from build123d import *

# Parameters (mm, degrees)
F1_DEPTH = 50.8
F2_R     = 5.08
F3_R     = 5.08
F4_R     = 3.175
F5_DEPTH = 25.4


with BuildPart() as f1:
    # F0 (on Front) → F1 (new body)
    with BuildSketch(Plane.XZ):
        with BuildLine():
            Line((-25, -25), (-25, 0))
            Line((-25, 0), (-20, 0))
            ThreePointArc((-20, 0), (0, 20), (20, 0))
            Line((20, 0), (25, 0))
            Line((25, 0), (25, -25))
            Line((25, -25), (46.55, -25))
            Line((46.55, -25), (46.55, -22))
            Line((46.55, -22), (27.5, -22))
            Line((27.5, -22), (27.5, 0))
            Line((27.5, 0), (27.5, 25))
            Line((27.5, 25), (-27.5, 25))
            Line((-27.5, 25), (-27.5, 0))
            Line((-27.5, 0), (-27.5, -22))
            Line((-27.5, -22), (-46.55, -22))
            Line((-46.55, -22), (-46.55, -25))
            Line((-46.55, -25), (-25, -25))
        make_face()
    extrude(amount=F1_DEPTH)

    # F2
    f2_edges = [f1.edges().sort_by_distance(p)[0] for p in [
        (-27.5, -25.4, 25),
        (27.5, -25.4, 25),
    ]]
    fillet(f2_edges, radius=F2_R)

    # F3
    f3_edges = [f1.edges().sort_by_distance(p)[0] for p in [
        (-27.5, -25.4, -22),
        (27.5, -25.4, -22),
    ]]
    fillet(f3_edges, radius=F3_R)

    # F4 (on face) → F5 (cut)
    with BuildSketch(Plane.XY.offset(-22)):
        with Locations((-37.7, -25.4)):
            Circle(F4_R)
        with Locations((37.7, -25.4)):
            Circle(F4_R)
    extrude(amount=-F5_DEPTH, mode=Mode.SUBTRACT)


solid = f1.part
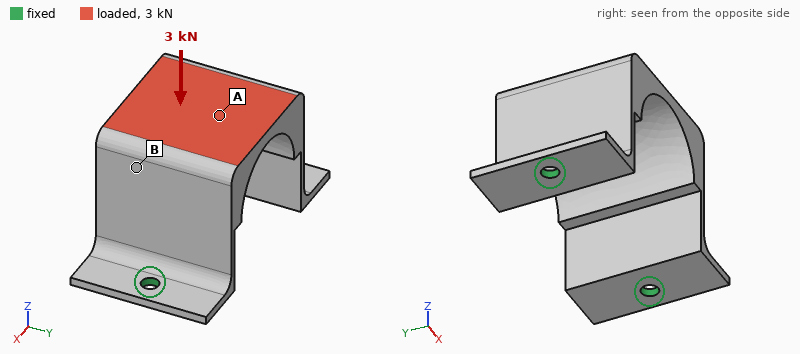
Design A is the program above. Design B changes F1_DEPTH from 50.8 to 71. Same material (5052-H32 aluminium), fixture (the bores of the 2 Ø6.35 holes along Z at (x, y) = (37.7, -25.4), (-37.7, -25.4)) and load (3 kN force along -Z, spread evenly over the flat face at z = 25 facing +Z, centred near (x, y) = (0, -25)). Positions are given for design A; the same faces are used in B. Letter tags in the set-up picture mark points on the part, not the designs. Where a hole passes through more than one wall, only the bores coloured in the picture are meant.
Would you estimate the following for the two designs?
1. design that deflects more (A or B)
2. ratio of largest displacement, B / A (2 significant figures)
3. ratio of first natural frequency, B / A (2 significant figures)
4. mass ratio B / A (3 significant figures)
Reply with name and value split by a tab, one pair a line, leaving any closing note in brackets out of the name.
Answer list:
design that deflects more	B
ratio of largest displacement, B / A	8.9
ratio of first natural frequency, B / A	0.78
mass ratio B / A	1.40
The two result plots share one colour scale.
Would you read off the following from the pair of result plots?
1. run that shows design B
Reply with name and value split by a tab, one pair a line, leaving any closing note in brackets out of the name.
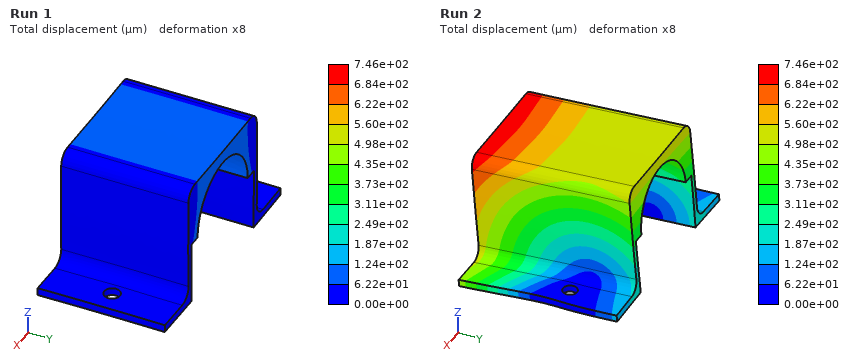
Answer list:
run that shows design B	Run 2
